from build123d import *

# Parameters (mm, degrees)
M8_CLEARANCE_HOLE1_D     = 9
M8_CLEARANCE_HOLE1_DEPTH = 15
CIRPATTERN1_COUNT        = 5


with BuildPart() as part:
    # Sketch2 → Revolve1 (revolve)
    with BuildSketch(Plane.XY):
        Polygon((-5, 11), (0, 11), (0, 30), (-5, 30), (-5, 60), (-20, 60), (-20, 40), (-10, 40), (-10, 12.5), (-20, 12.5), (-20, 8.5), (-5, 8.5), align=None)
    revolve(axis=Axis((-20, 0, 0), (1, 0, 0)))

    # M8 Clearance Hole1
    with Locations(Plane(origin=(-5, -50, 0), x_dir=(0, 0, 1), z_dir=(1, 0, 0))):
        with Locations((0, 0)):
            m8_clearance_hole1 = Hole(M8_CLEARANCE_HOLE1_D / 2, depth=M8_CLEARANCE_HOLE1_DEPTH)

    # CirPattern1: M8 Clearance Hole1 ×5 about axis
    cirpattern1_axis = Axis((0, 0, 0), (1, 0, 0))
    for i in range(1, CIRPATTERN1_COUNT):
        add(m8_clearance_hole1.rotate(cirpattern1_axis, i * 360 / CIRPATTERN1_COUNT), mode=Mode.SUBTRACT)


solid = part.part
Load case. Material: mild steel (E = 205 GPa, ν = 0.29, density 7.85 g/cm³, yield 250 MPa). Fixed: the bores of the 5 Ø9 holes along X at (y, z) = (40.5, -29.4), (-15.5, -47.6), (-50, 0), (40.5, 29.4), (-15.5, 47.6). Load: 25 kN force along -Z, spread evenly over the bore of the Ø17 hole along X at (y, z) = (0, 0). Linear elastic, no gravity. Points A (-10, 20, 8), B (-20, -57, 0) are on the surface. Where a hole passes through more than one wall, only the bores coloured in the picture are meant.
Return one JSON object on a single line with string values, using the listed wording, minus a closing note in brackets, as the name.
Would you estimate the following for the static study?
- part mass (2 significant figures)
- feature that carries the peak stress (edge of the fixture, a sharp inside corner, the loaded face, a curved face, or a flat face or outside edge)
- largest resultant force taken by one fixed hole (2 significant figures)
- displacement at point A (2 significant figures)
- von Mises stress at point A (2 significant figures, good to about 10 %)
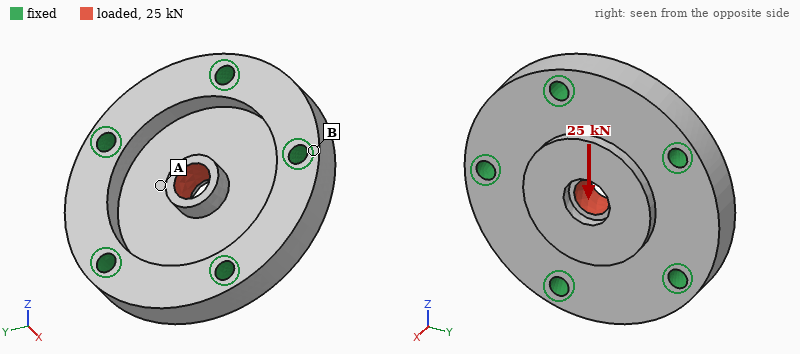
{"part mass": "1.0 kg", "feature that carries the peak stress": "the loaded face", "largest resultant force taken by one fixed hole": "6.1 kN", "displacement at point A": "8.3 µm", "von Mises stress at point A": "65 MPa"}
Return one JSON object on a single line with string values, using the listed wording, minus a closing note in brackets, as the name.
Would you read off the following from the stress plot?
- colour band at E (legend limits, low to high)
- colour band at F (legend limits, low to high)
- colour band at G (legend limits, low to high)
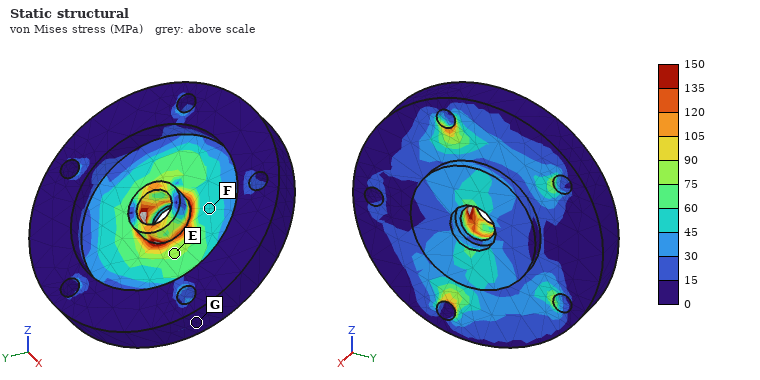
{"colour band at E": "75 to 90 MPa", "colour band at F": "45 to 60 MPa", "colour band at G": "0 to 15 MPa"}
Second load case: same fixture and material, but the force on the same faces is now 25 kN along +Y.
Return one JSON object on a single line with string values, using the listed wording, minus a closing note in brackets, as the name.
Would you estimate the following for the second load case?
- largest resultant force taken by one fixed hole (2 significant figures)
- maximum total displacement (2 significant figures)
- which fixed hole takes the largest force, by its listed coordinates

{"largest resultant force taken by one fixed hole": "6.3 kN", "maximum total displacement": "38 µm", "which fixed hole takes the largest force, by its listed coordinates": "(-50, 0)"}
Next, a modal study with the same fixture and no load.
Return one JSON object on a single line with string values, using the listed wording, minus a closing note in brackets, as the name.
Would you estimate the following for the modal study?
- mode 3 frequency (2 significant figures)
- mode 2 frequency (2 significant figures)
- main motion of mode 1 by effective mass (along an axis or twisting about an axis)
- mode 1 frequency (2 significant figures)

{"mode 3 frequency": "13 kHz", "mode 2 frequency": "13 kHz", "main motion of mode 1 by effective mass": "along X", "mode 1 frequency": "7900 Hz"}
